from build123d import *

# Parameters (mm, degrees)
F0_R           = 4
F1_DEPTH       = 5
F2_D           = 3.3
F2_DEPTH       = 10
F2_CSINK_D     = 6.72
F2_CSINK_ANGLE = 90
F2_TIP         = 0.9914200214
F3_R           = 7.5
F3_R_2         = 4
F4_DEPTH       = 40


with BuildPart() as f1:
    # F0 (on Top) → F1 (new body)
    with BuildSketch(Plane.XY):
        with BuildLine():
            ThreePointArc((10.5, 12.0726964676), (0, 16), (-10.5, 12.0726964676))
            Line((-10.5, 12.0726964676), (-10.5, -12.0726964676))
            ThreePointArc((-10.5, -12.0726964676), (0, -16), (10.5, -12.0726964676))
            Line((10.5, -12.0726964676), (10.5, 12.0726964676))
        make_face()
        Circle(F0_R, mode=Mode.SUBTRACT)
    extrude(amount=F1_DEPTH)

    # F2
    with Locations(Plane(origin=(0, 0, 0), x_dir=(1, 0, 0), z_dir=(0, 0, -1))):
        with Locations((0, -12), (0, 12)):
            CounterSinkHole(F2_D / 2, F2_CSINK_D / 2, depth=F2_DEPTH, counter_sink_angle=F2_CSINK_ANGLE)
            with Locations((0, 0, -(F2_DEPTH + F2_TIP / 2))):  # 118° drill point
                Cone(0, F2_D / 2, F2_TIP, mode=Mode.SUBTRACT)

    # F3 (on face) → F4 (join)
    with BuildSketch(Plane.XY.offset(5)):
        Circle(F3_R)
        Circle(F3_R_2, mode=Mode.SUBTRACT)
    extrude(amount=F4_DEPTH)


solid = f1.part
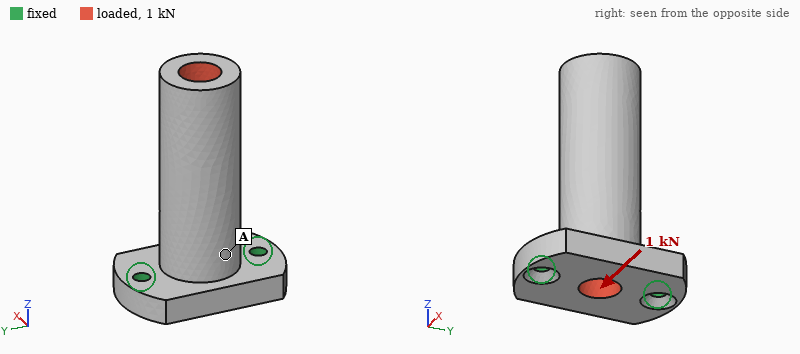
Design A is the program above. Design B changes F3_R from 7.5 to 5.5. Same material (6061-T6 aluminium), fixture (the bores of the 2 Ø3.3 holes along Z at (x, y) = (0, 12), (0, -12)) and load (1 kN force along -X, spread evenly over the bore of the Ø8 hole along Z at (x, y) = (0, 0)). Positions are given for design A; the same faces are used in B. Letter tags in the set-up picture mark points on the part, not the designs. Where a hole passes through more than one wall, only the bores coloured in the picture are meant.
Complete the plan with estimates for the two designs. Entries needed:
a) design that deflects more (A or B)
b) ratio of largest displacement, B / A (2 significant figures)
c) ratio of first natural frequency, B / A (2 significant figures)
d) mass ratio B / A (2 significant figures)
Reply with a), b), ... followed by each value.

a) B
b) 1.8
c) 1.3
d) 0.58
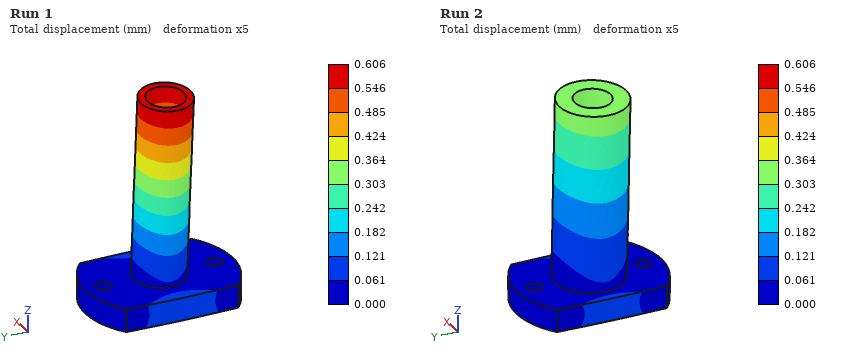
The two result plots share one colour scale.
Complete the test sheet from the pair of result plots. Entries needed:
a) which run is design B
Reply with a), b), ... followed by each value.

a) Run 1
